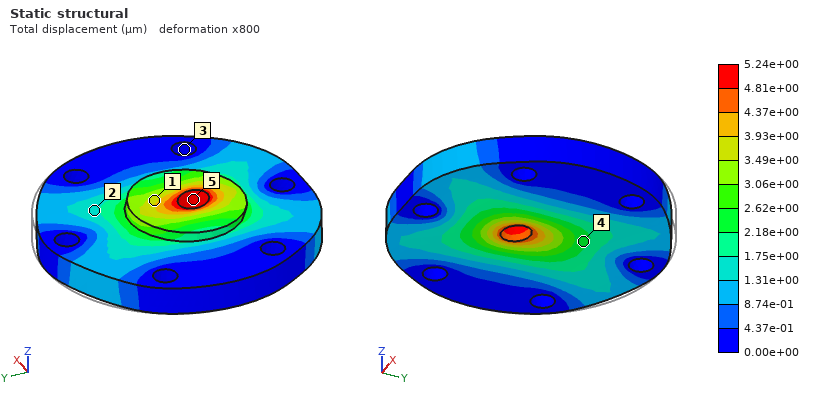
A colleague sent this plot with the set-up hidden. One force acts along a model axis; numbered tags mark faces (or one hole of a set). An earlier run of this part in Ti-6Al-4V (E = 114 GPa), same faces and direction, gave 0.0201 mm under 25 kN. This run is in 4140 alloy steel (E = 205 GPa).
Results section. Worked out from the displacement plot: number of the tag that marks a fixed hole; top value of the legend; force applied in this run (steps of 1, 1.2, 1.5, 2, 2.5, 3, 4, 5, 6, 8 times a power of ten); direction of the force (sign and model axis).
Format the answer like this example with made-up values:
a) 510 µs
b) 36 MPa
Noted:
a) 3
b) 5.24e+00 µm
c) 12 kN
d) -Y
